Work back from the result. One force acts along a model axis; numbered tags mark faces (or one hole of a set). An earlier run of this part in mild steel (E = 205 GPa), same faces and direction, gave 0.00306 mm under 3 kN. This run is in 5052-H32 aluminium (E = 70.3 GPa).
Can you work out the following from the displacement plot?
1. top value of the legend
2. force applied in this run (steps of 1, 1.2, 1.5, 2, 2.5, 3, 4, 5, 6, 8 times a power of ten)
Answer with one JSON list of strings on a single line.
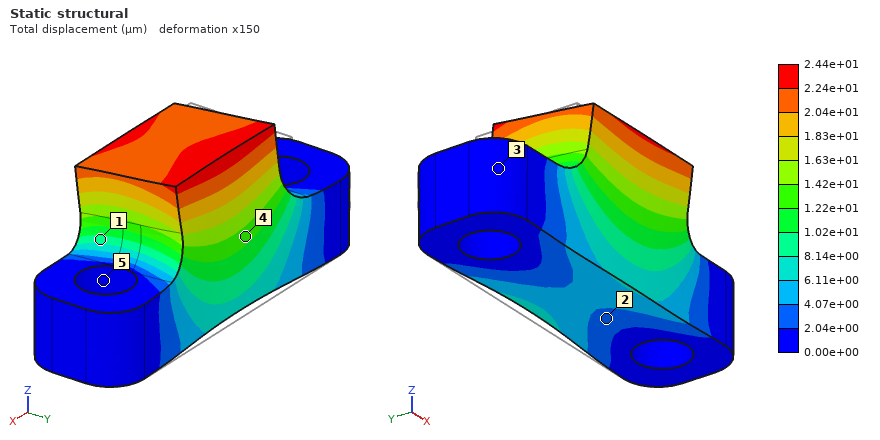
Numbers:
["2.44e+01 µm", "8 kN"]
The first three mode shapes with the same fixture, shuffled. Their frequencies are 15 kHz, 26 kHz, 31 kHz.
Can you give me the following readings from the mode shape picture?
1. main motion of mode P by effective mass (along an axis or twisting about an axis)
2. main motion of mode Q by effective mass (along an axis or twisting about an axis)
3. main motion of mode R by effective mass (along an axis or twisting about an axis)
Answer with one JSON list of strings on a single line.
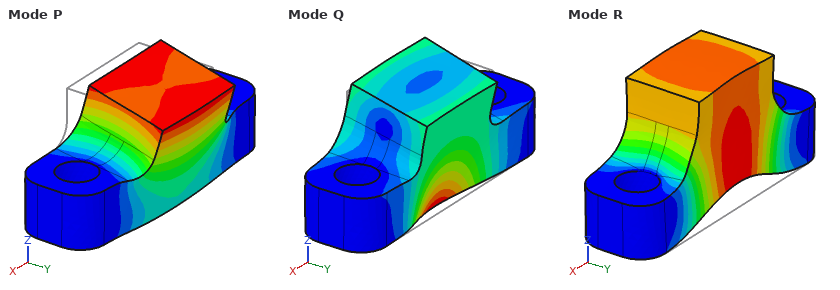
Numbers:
["along Y", "along Y", "along Z"]
